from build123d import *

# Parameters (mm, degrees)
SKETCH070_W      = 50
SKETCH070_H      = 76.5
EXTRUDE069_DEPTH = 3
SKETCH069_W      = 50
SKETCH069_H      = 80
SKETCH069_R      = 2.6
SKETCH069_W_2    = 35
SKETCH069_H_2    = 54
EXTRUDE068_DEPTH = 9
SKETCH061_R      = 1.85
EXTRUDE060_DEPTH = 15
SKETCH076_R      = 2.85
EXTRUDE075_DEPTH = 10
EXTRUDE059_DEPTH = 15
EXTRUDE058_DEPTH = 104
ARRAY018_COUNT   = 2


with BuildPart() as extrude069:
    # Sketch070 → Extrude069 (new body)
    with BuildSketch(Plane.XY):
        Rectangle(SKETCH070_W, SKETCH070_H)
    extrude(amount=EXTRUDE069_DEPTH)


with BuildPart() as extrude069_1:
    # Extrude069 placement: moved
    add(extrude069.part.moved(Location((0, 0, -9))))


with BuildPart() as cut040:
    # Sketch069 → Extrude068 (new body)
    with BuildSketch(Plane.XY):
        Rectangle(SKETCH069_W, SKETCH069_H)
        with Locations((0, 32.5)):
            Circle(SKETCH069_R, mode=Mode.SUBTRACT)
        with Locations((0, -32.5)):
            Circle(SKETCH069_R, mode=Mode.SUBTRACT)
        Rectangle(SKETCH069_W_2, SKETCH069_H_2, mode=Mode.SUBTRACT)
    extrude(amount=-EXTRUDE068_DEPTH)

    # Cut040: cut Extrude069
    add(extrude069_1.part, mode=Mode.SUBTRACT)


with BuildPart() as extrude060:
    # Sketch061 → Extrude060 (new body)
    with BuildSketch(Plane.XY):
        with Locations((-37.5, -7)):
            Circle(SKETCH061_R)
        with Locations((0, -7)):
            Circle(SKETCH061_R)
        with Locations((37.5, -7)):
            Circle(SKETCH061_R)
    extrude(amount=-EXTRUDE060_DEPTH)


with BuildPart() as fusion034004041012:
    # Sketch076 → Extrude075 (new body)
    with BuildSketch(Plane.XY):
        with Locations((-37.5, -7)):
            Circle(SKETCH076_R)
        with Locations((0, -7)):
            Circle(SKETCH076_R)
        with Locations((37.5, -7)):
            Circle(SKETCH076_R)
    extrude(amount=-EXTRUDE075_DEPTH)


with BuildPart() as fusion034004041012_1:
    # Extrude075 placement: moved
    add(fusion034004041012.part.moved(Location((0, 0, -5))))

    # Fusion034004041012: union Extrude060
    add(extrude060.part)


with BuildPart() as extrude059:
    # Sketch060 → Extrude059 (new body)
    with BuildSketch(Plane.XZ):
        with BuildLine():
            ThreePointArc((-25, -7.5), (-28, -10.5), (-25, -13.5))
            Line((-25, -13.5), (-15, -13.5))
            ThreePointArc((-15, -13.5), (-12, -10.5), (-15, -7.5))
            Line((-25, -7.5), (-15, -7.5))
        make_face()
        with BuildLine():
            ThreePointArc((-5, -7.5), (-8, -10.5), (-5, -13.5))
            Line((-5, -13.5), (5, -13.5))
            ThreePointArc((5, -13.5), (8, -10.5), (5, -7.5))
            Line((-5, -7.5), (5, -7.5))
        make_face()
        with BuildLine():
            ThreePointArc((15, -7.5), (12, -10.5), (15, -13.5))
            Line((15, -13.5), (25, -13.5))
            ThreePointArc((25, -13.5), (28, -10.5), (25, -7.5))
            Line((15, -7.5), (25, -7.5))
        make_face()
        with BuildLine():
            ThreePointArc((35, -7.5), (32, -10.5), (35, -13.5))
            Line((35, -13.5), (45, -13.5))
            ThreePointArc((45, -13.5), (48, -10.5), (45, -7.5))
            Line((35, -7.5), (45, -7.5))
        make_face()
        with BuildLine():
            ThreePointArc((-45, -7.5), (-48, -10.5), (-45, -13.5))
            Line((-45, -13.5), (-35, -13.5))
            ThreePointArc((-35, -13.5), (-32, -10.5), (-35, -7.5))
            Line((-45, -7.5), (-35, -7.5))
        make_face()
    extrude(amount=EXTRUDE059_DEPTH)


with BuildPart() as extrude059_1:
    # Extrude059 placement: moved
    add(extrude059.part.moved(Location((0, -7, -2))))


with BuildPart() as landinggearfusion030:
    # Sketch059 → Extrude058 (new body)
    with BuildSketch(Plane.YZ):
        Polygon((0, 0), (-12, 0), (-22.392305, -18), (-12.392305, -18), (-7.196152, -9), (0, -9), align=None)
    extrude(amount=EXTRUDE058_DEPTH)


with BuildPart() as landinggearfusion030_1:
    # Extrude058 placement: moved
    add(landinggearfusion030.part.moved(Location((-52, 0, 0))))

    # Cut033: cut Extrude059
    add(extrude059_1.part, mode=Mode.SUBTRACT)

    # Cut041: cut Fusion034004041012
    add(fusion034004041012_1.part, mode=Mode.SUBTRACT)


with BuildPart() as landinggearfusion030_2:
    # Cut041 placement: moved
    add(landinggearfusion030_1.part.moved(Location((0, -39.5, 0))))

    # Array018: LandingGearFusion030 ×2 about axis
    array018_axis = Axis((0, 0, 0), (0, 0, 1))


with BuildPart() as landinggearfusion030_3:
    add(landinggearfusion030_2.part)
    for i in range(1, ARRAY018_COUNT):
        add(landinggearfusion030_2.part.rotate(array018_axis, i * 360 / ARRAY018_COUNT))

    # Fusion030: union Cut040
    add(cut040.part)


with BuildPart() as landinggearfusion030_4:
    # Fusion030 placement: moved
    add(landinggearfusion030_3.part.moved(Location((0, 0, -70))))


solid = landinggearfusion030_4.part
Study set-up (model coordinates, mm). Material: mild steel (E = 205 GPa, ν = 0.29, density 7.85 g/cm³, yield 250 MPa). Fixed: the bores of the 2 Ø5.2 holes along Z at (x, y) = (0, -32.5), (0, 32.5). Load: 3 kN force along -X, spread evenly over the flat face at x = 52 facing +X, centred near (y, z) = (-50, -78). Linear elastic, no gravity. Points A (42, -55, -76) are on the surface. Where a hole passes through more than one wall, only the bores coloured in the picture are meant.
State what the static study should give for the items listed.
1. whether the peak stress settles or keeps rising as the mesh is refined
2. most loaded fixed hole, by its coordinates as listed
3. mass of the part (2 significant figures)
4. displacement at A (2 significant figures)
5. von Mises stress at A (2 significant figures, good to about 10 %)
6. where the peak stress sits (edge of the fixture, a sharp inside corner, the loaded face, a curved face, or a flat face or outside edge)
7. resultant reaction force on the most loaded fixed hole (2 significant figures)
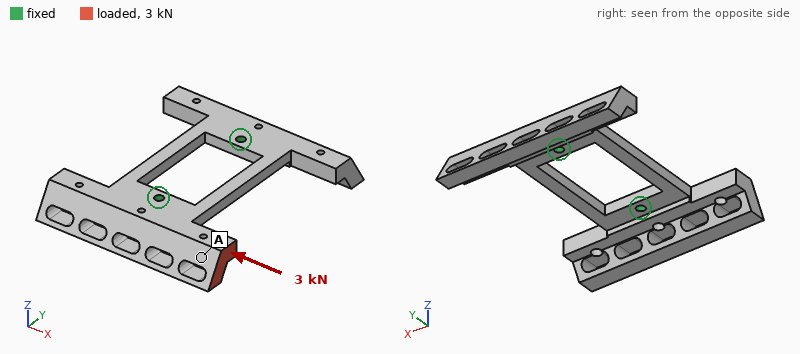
keeps rising
(0, -32.5)
380 g
59 µm
24 MPa
edge of the fixture
3.2 kN
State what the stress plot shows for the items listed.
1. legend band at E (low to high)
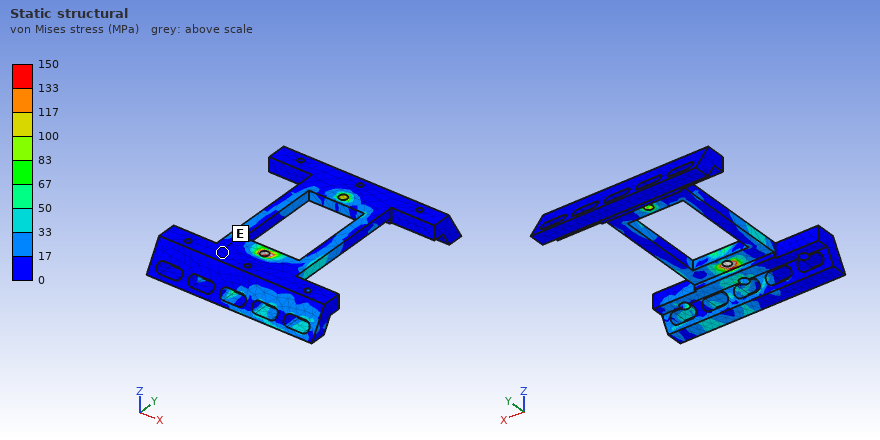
0 to 17 MPa
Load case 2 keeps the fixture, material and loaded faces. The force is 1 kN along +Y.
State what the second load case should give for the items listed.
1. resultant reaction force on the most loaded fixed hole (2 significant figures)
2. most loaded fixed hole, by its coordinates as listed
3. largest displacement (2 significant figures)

640 N
(0, -32.5)
0.11 mm
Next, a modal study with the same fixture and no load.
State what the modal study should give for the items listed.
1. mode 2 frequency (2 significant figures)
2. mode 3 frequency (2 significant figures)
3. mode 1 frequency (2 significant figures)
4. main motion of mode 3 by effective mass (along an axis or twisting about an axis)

1600 Hz
2400 Hz
1600 Hz
twisting about Z
